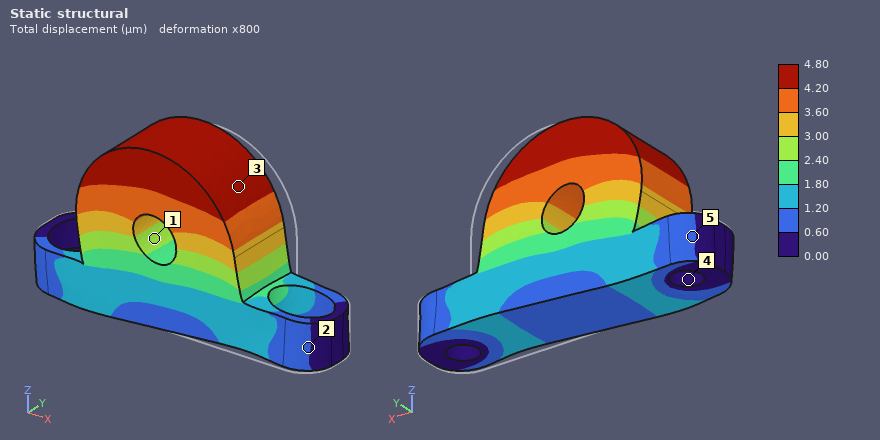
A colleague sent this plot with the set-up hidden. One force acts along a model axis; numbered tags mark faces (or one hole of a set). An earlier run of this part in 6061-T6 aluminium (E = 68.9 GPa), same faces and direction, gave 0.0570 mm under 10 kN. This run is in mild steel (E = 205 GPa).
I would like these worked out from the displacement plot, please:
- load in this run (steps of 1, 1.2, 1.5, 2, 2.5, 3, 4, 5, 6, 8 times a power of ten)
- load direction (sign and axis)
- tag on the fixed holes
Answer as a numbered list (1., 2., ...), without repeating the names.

1. 2.5 kN
2. -X
3. 4
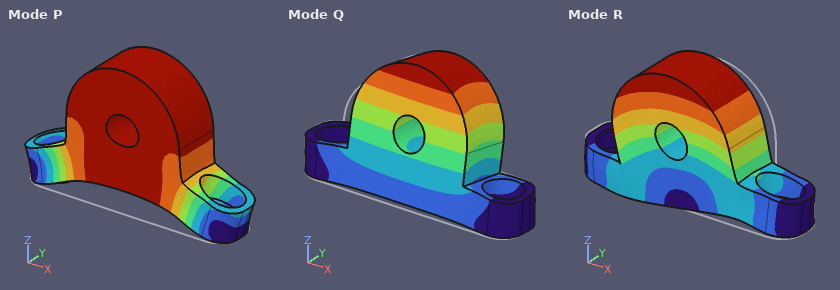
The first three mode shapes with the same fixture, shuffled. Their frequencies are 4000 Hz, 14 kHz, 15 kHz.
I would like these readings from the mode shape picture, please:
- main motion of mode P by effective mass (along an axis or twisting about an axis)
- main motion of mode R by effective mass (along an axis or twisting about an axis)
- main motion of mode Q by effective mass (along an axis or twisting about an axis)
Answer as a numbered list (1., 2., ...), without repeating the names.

1. along Z
2. along X
3. along Y
